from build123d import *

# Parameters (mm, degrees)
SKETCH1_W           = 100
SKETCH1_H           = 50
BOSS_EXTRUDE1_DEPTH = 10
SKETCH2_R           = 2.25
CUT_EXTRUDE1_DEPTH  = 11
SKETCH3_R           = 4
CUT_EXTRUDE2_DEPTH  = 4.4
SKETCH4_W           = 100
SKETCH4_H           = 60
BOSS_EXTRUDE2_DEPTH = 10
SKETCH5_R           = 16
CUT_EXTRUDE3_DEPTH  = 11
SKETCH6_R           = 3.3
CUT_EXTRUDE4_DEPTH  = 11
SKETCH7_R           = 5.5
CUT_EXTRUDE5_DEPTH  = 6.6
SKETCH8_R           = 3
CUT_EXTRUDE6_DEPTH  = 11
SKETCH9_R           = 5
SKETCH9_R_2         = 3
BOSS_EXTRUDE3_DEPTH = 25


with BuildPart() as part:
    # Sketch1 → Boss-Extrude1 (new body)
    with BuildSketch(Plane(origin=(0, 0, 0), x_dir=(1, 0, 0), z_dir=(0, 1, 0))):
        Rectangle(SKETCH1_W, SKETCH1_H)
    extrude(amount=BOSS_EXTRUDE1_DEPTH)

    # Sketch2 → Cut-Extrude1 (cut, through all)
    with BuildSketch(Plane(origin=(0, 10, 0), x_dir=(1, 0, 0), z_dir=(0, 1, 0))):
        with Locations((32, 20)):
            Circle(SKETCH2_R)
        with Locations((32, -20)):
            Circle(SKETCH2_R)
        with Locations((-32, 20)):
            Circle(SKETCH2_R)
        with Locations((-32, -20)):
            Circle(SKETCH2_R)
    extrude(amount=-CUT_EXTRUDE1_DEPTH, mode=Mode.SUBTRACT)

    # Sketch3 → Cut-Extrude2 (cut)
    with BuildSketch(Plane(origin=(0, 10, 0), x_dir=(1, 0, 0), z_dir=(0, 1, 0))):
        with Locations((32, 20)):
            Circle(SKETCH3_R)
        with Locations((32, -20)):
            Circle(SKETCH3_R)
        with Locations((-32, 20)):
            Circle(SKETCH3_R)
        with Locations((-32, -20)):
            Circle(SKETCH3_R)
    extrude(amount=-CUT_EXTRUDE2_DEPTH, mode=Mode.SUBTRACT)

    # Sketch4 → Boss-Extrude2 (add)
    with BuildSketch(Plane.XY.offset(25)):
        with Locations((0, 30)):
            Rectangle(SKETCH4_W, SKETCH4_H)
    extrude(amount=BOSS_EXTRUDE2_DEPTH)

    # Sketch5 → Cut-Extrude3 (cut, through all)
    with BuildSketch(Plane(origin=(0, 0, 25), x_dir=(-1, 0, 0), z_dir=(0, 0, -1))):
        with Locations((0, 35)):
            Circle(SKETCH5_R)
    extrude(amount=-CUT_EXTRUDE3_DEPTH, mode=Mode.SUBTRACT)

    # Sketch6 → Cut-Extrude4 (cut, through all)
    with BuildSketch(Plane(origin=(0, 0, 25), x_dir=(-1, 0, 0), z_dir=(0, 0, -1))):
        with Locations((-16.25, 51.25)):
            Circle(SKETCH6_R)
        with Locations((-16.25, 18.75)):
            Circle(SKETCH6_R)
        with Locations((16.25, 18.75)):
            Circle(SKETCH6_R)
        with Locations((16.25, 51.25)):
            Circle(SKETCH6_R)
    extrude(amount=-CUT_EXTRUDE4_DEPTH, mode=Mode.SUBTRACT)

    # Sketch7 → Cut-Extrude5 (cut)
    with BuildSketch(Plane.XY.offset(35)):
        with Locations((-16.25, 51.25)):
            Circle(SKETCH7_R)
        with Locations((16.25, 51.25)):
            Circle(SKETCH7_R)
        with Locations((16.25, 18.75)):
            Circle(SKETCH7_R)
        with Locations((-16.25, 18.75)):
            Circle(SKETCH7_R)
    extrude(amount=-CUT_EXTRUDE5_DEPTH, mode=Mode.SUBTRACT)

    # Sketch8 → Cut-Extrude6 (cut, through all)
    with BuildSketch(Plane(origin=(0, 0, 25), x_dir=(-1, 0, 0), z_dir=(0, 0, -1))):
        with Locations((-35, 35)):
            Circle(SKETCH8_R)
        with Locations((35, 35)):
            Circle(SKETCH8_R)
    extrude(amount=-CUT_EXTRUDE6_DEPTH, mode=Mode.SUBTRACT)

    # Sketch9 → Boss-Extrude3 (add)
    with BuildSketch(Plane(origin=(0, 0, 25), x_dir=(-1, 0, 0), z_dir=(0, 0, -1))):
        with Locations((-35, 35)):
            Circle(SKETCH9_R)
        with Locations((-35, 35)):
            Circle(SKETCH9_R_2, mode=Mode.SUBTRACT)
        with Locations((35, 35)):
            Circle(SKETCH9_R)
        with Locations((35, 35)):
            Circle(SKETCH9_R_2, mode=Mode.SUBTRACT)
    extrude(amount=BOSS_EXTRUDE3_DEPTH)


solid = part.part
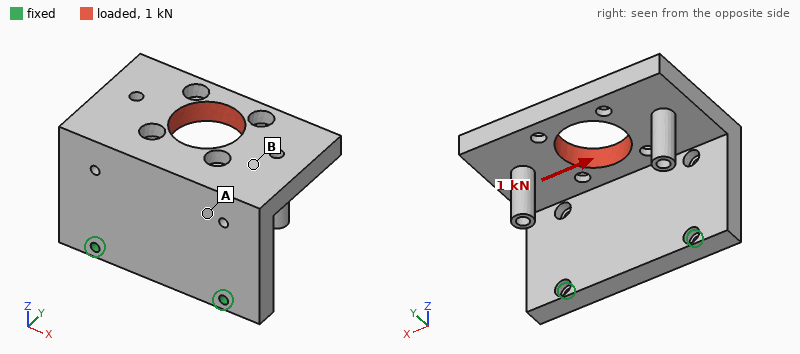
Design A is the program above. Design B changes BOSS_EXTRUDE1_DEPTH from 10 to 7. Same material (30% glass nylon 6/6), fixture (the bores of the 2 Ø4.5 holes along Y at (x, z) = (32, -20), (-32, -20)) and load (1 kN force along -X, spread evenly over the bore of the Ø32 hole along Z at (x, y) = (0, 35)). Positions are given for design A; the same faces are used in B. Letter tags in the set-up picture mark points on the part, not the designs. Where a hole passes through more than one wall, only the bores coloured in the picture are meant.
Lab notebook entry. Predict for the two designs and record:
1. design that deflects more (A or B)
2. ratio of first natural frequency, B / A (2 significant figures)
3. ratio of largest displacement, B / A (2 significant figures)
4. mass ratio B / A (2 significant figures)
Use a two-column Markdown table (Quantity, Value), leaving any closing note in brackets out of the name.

| Quantity | Value |
|---|---|
| design that deflects more | B |
| ratio of first natural frequency, B / A | 0.78 |
| ratio of largest displacement, B / A | 2.0 |
| mass ratio B / A | 0.86 |
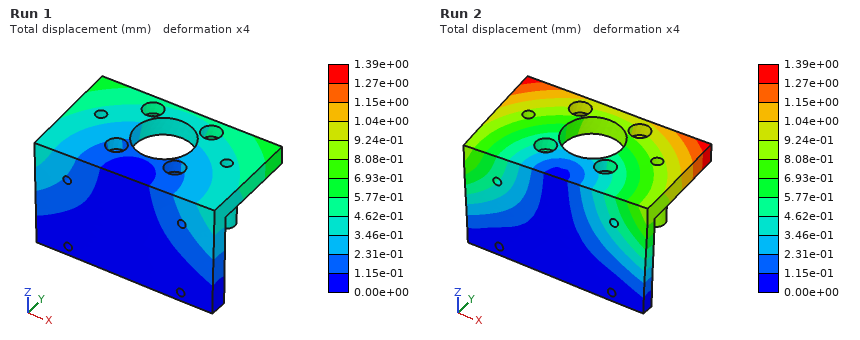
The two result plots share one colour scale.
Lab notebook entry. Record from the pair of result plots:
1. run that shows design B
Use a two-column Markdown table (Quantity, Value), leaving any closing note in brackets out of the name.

| Quantity | Value |
|---|---|
| run that shows design B | Run 2 |
